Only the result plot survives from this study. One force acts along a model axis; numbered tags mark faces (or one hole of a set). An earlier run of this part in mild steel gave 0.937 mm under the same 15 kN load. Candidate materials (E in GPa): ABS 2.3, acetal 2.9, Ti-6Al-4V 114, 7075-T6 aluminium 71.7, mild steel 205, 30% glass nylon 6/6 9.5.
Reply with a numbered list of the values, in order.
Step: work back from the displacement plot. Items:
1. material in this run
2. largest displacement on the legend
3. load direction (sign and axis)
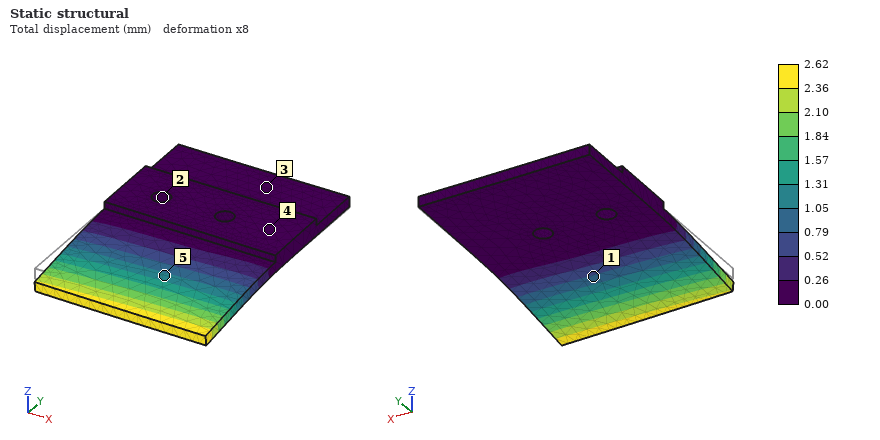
1. 7075-T6 aluminium
2. 2.62 mm
3. -Z
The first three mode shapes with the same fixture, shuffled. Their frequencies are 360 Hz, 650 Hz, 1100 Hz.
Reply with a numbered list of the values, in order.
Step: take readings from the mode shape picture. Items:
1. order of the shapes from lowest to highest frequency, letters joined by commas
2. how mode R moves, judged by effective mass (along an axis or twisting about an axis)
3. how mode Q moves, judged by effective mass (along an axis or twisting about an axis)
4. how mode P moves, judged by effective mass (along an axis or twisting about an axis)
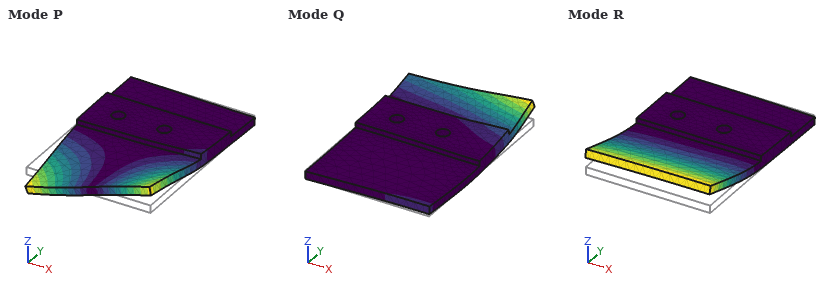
1. R, P, Q
2. along Z
3. along Z
4. twisting about Y
